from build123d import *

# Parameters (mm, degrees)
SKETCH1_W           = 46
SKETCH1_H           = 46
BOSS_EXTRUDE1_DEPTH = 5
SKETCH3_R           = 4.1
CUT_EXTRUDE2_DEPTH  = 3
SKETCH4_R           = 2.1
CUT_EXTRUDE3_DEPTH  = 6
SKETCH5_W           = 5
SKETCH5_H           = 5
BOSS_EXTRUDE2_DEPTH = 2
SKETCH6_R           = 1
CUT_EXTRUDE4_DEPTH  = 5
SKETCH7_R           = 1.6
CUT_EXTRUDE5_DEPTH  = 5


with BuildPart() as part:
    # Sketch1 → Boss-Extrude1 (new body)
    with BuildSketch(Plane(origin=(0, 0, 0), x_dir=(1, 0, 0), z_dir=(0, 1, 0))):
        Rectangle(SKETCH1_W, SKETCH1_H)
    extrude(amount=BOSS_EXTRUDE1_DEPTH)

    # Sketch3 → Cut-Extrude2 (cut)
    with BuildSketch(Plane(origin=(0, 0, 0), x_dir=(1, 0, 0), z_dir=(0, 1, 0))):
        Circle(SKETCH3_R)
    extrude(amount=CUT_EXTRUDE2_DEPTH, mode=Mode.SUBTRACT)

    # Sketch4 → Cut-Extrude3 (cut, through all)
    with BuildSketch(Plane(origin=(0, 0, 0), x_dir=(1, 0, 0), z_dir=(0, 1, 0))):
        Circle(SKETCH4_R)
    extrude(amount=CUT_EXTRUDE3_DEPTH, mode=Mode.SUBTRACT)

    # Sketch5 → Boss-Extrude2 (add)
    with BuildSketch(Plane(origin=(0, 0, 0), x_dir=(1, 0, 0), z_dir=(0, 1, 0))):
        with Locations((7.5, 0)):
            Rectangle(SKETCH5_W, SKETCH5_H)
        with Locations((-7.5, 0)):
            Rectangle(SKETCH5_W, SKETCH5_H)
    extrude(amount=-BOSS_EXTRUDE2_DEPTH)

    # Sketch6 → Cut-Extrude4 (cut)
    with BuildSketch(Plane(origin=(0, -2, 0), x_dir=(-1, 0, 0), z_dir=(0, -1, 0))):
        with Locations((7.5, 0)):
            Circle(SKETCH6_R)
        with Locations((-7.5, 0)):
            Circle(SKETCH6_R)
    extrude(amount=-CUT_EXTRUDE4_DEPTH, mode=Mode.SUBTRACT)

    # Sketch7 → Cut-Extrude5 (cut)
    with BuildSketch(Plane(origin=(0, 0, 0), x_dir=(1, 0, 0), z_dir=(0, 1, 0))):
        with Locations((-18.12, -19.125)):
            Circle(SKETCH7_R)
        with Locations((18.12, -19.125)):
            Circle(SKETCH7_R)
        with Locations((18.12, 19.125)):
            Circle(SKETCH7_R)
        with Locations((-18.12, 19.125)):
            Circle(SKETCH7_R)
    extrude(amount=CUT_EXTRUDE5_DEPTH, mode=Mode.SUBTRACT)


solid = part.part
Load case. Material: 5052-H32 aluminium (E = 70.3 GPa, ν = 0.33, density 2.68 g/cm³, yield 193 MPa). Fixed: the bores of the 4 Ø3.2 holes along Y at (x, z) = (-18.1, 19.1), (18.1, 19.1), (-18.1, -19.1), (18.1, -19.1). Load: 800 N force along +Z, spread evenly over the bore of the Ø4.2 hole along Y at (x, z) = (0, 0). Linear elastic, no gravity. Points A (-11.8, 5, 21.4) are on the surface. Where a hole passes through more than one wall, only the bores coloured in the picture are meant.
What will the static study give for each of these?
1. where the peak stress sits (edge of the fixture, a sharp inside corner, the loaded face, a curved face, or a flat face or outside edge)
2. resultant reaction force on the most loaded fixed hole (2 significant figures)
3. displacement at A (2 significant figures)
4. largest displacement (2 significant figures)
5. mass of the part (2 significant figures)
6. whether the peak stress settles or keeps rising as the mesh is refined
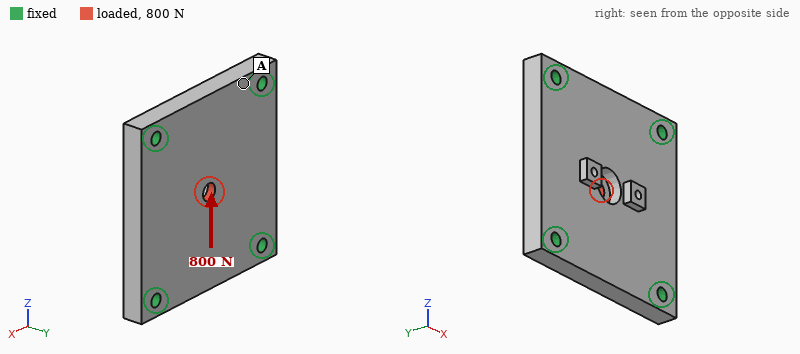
a sharp inside corner
230 N
0.64 µm
3.4 µm
28 g
keeps rising
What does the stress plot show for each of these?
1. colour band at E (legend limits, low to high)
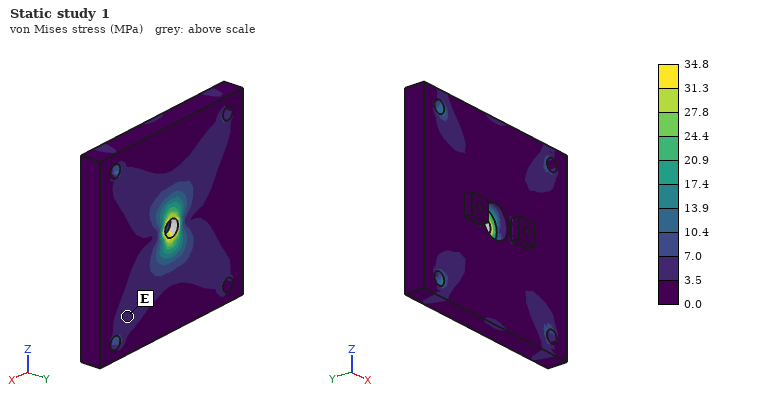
3.5 to 7.0 MPa
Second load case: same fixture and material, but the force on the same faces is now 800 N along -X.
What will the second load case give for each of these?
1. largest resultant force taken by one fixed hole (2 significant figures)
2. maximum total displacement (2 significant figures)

230 N
3.5 µm
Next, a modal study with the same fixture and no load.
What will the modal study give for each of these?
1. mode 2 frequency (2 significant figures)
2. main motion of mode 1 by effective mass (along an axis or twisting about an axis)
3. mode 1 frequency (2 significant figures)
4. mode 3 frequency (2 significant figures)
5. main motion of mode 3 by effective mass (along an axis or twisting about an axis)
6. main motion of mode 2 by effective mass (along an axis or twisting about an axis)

18 kHz
along Y
12 kHz
20 kHz
twisting about X
twisting about Z
